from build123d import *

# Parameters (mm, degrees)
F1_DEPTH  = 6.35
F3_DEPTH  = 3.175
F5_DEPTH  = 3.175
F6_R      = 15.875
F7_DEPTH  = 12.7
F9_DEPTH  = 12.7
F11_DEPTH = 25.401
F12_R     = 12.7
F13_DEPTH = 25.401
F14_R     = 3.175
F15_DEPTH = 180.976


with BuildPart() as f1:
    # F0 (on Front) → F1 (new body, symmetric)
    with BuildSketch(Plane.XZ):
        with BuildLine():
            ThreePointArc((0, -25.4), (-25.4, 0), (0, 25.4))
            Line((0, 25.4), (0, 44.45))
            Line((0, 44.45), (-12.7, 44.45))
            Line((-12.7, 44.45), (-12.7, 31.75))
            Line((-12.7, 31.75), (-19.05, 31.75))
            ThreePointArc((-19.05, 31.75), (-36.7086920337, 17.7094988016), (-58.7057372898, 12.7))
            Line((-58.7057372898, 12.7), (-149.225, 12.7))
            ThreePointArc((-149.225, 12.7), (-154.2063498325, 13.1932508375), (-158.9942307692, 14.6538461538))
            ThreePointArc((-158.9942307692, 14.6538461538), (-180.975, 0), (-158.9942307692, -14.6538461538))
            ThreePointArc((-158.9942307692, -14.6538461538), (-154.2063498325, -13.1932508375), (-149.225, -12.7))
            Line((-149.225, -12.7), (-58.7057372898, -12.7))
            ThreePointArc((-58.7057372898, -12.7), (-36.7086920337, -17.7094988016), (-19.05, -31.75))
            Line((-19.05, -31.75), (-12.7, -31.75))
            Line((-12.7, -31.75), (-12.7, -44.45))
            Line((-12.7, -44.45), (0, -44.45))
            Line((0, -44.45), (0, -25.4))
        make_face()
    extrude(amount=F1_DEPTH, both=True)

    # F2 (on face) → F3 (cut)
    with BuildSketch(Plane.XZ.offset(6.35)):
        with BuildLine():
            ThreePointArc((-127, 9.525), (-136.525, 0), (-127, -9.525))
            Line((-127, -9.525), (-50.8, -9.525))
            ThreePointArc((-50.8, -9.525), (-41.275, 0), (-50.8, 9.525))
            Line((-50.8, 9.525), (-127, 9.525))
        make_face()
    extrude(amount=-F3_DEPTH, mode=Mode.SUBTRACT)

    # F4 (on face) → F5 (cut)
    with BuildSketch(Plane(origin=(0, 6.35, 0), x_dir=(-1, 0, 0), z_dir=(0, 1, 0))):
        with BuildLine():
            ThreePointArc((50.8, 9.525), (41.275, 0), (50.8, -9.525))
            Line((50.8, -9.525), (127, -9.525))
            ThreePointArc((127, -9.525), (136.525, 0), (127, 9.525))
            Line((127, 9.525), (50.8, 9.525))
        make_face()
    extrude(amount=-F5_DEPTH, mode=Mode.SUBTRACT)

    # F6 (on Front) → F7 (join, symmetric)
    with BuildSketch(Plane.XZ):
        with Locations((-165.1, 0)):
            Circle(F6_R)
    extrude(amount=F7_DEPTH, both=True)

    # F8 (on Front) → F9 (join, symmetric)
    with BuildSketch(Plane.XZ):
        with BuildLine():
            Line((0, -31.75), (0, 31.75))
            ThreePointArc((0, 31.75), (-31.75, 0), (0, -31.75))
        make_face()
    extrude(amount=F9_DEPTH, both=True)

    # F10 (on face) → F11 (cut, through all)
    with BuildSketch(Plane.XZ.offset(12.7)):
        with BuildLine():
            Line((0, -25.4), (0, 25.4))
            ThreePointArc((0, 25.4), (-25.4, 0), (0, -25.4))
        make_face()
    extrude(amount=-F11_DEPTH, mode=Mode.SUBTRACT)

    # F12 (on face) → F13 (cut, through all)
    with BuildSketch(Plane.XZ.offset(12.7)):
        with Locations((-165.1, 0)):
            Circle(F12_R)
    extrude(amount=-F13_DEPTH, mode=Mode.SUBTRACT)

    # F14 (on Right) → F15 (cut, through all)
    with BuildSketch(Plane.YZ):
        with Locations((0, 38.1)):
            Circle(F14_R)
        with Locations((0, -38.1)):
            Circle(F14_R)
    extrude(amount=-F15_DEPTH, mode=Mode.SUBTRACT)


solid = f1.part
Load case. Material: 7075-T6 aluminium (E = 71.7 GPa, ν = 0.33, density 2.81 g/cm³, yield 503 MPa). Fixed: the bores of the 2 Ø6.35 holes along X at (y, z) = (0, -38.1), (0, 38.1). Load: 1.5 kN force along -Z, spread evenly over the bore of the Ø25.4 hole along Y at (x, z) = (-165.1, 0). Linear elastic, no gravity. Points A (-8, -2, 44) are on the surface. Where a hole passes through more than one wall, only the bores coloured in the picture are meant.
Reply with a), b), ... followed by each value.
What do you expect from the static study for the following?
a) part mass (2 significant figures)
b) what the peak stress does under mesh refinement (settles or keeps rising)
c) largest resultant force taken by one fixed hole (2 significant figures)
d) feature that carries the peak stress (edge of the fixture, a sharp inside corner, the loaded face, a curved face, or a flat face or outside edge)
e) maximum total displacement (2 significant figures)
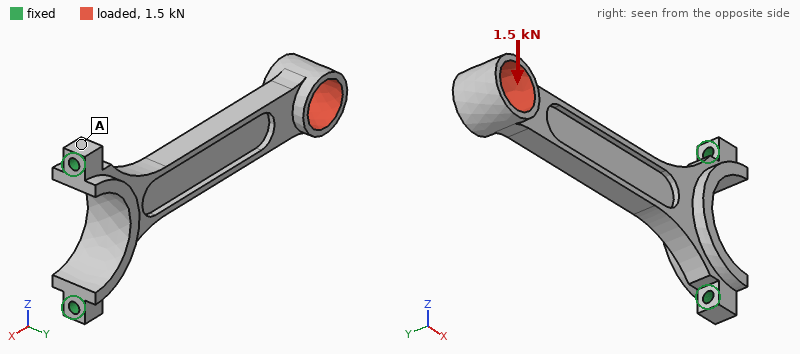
a) 160 g
b) keeps rising
c) 4.3 kN
d) edge of the fixture
e) 1.6 mm
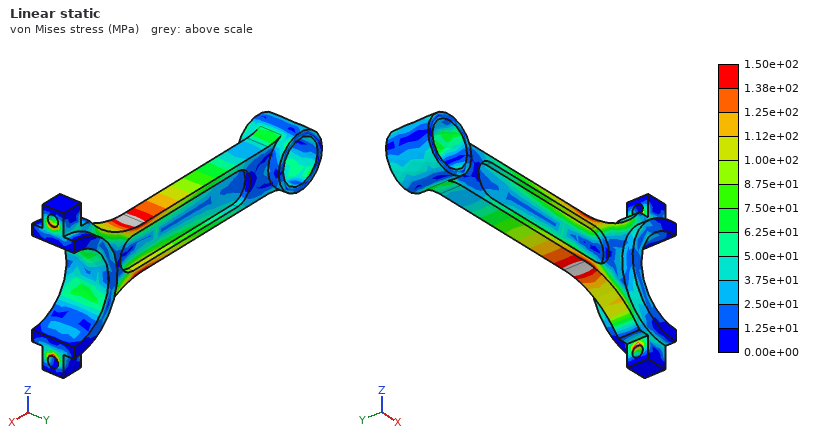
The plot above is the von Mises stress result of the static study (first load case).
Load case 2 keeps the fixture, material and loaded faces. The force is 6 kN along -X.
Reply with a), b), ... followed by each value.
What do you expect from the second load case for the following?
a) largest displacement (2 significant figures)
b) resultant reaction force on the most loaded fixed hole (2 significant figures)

a) 0.12 mm
b) 3.8 kN
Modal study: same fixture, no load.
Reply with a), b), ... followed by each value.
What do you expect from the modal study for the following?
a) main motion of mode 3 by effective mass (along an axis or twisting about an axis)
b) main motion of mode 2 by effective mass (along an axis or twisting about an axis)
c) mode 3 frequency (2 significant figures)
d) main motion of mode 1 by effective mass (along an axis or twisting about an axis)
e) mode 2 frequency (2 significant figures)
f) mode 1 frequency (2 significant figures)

a) along Y
b) along Z
c) 1700 Hz
d) along Y
e) 900 Hz
f) 300 Hz
